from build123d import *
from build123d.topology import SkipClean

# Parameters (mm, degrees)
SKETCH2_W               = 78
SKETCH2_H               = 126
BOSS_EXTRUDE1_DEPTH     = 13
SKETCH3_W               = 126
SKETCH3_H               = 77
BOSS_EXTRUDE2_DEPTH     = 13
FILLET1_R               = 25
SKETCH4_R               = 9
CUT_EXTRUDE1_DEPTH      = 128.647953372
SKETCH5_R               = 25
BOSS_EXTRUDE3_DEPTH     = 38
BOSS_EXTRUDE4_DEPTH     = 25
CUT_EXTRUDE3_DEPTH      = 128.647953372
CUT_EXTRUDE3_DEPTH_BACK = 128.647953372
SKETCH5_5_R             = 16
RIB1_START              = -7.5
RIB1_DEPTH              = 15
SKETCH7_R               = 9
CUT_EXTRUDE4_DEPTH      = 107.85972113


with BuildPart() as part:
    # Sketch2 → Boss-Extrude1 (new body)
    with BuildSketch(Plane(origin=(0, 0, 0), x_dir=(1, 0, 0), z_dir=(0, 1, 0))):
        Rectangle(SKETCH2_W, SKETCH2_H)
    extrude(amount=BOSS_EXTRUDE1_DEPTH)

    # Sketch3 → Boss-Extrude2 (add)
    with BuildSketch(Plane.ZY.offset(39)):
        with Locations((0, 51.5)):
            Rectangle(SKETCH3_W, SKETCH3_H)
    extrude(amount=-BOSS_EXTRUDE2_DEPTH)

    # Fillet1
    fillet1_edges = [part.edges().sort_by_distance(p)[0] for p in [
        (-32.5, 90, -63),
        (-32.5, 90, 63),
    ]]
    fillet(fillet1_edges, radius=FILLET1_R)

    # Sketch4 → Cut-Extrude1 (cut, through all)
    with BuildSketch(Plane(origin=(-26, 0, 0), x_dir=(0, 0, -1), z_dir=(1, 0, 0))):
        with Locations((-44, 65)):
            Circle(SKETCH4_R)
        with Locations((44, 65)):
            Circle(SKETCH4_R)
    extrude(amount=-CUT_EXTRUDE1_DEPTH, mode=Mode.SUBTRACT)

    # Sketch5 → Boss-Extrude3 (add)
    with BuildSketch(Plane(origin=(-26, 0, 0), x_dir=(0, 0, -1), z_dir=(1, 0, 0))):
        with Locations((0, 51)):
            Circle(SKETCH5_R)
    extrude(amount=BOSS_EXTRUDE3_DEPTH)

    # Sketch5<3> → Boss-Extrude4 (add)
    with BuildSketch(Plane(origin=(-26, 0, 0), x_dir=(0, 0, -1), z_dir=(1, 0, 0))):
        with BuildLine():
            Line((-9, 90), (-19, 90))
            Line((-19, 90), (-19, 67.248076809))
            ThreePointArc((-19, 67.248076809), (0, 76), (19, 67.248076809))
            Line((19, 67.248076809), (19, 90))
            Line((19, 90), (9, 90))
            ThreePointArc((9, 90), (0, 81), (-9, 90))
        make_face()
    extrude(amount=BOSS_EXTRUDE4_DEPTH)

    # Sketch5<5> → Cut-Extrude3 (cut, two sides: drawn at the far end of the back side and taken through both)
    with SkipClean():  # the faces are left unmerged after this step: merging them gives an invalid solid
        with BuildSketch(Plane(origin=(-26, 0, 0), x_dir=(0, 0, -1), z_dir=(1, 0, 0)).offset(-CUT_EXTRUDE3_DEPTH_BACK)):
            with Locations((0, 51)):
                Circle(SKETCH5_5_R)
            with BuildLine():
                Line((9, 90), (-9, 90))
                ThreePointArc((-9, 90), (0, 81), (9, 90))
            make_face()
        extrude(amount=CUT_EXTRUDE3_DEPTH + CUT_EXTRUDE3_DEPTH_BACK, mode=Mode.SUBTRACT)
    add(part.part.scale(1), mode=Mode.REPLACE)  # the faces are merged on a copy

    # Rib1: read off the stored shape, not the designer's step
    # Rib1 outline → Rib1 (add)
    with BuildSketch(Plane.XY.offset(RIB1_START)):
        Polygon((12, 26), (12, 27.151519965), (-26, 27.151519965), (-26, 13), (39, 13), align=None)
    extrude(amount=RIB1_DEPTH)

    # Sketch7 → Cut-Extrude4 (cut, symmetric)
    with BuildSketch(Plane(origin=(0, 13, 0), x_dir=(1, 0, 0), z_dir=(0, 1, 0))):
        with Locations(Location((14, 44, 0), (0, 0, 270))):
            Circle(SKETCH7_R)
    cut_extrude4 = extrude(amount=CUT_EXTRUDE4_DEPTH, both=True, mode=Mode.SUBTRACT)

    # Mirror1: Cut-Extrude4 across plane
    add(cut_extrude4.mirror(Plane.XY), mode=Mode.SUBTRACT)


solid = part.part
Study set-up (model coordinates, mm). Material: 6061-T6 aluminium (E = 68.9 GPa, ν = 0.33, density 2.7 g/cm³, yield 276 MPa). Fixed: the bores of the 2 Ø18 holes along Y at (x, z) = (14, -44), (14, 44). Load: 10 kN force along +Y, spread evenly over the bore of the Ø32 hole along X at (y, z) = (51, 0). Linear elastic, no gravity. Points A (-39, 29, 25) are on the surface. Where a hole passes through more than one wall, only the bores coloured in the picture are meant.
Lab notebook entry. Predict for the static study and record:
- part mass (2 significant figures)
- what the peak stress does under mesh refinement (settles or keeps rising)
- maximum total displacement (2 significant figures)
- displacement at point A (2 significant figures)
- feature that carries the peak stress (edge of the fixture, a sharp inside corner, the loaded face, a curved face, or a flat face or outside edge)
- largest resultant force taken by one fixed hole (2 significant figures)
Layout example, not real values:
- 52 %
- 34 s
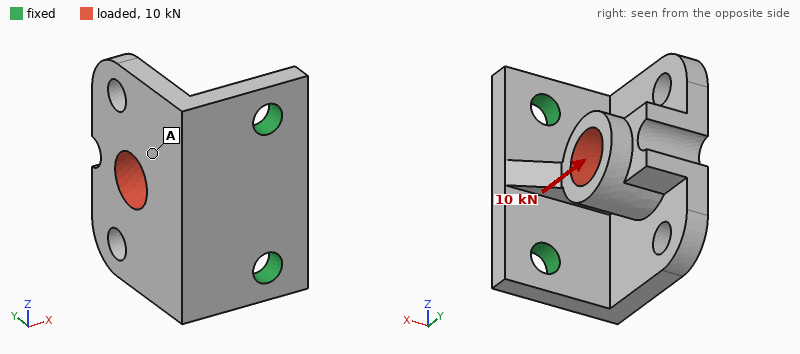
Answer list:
- 790 g
- keeps rising
- 0.15 mm
- 0.11 mm
- edge of the fixture
- 5.0 kN
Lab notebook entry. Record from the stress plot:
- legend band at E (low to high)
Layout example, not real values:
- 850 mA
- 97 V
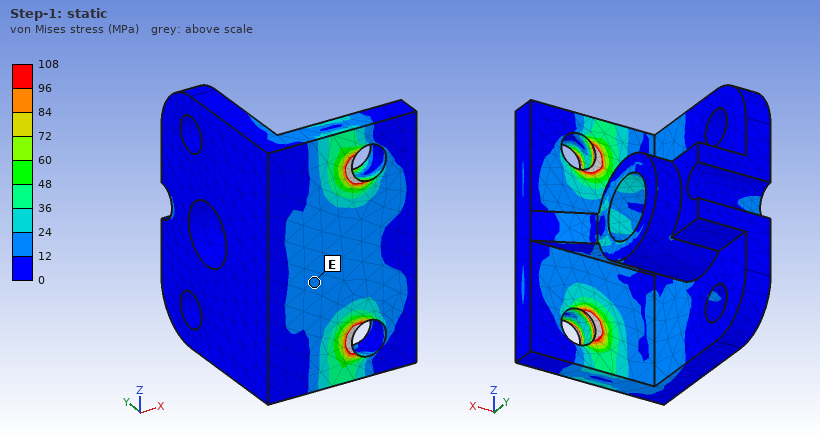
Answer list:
- 12 to 24 MPa
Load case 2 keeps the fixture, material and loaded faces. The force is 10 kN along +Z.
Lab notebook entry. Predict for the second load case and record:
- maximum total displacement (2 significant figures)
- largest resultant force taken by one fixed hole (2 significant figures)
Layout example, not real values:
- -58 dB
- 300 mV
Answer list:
- 0.16 mm
- 7.9 kN
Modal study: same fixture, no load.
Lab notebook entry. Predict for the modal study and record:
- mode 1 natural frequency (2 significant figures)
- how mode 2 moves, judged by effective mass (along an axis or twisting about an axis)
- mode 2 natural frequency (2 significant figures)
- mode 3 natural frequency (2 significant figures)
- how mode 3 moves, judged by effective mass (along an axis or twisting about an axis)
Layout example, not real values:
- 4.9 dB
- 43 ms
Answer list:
- 1200 Hz
- along Z
- 2000 Hz
- 3500 Hz
- along Y
